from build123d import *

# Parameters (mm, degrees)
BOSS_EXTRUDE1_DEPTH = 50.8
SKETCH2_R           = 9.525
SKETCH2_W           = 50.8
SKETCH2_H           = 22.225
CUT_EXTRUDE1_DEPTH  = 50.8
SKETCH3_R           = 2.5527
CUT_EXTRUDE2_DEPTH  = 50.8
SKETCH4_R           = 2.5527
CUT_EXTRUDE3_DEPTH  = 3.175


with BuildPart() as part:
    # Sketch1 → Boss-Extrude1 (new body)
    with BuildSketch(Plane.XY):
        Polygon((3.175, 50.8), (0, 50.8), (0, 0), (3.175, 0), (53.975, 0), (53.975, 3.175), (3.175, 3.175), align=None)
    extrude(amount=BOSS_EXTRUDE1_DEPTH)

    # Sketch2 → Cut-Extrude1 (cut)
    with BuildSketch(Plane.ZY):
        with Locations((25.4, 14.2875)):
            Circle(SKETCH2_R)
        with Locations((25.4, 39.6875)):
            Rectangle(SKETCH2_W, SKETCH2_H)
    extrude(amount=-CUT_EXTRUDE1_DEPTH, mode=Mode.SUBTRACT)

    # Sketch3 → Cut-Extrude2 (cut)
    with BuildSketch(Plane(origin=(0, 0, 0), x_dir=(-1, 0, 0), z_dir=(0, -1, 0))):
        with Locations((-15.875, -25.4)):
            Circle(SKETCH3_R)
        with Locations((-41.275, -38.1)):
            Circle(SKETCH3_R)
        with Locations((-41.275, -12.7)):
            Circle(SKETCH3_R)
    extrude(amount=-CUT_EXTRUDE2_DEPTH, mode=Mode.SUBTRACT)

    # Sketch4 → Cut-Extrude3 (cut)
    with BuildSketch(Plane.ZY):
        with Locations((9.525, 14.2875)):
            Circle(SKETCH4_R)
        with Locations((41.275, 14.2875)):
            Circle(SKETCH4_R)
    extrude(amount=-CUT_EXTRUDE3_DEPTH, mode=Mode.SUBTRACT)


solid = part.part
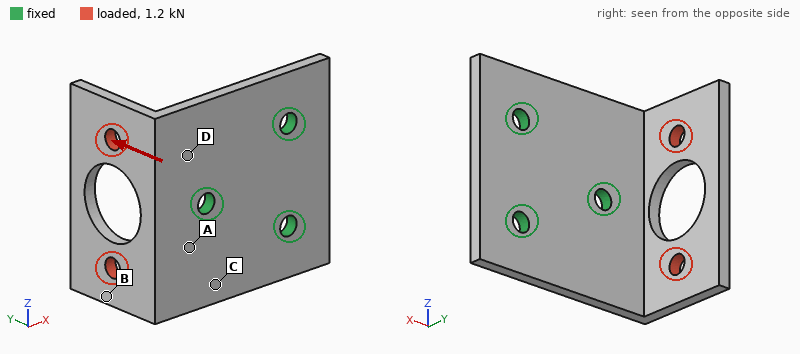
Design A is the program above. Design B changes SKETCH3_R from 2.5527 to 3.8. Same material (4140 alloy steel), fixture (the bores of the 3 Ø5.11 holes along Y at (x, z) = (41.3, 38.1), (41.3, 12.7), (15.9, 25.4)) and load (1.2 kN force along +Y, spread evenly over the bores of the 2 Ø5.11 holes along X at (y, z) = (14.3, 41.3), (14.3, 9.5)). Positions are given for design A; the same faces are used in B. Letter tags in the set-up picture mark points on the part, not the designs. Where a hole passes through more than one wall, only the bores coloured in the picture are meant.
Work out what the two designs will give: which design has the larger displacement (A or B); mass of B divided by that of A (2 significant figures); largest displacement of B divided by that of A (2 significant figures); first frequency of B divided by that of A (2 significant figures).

A
0.98
0.79
1.0
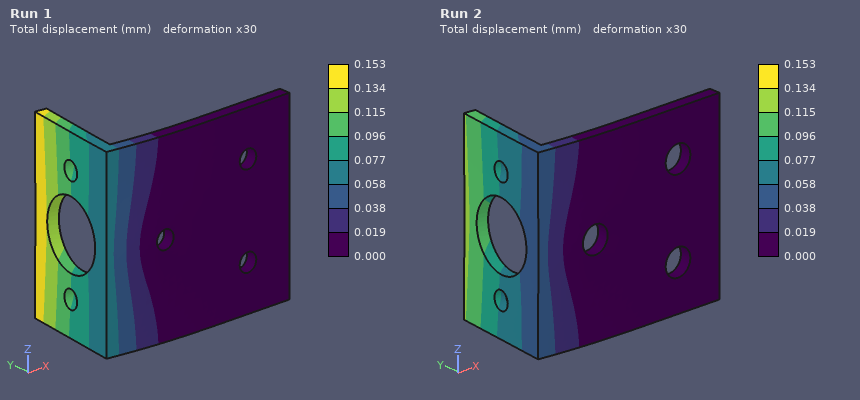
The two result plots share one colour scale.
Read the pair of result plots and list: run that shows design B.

Run 2
